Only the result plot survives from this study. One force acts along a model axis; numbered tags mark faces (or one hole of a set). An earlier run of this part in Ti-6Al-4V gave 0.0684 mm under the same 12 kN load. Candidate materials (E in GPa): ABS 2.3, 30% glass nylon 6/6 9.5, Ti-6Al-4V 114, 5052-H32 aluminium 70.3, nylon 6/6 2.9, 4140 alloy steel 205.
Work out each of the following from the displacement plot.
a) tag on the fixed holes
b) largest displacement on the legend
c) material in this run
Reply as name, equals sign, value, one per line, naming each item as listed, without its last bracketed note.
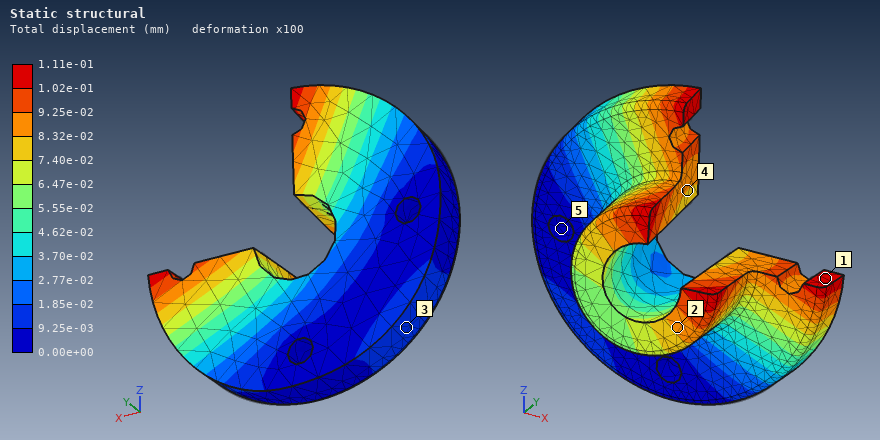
tag on the fixed holes = 5
largest displacement on the legend = 1.11e-01 mm
material in this run = 5052-H32 aluminium
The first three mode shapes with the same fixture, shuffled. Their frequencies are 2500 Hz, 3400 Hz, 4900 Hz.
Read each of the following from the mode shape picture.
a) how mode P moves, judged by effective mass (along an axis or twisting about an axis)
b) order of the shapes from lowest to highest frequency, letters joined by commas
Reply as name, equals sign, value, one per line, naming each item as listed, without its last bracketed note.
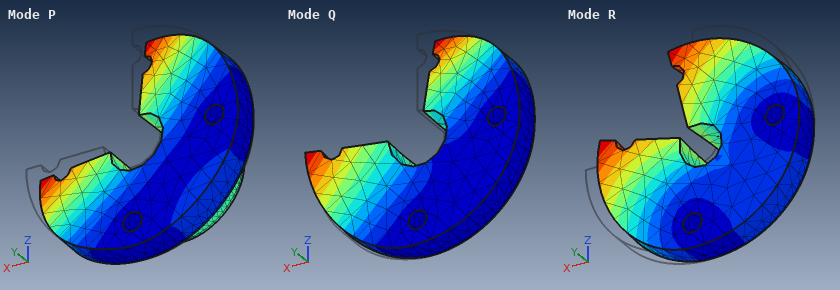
how mode P moves, judged by effective mass = along Y
order of the shapes from lowest to highest frequency, letters joined by commas = P, Q, R
